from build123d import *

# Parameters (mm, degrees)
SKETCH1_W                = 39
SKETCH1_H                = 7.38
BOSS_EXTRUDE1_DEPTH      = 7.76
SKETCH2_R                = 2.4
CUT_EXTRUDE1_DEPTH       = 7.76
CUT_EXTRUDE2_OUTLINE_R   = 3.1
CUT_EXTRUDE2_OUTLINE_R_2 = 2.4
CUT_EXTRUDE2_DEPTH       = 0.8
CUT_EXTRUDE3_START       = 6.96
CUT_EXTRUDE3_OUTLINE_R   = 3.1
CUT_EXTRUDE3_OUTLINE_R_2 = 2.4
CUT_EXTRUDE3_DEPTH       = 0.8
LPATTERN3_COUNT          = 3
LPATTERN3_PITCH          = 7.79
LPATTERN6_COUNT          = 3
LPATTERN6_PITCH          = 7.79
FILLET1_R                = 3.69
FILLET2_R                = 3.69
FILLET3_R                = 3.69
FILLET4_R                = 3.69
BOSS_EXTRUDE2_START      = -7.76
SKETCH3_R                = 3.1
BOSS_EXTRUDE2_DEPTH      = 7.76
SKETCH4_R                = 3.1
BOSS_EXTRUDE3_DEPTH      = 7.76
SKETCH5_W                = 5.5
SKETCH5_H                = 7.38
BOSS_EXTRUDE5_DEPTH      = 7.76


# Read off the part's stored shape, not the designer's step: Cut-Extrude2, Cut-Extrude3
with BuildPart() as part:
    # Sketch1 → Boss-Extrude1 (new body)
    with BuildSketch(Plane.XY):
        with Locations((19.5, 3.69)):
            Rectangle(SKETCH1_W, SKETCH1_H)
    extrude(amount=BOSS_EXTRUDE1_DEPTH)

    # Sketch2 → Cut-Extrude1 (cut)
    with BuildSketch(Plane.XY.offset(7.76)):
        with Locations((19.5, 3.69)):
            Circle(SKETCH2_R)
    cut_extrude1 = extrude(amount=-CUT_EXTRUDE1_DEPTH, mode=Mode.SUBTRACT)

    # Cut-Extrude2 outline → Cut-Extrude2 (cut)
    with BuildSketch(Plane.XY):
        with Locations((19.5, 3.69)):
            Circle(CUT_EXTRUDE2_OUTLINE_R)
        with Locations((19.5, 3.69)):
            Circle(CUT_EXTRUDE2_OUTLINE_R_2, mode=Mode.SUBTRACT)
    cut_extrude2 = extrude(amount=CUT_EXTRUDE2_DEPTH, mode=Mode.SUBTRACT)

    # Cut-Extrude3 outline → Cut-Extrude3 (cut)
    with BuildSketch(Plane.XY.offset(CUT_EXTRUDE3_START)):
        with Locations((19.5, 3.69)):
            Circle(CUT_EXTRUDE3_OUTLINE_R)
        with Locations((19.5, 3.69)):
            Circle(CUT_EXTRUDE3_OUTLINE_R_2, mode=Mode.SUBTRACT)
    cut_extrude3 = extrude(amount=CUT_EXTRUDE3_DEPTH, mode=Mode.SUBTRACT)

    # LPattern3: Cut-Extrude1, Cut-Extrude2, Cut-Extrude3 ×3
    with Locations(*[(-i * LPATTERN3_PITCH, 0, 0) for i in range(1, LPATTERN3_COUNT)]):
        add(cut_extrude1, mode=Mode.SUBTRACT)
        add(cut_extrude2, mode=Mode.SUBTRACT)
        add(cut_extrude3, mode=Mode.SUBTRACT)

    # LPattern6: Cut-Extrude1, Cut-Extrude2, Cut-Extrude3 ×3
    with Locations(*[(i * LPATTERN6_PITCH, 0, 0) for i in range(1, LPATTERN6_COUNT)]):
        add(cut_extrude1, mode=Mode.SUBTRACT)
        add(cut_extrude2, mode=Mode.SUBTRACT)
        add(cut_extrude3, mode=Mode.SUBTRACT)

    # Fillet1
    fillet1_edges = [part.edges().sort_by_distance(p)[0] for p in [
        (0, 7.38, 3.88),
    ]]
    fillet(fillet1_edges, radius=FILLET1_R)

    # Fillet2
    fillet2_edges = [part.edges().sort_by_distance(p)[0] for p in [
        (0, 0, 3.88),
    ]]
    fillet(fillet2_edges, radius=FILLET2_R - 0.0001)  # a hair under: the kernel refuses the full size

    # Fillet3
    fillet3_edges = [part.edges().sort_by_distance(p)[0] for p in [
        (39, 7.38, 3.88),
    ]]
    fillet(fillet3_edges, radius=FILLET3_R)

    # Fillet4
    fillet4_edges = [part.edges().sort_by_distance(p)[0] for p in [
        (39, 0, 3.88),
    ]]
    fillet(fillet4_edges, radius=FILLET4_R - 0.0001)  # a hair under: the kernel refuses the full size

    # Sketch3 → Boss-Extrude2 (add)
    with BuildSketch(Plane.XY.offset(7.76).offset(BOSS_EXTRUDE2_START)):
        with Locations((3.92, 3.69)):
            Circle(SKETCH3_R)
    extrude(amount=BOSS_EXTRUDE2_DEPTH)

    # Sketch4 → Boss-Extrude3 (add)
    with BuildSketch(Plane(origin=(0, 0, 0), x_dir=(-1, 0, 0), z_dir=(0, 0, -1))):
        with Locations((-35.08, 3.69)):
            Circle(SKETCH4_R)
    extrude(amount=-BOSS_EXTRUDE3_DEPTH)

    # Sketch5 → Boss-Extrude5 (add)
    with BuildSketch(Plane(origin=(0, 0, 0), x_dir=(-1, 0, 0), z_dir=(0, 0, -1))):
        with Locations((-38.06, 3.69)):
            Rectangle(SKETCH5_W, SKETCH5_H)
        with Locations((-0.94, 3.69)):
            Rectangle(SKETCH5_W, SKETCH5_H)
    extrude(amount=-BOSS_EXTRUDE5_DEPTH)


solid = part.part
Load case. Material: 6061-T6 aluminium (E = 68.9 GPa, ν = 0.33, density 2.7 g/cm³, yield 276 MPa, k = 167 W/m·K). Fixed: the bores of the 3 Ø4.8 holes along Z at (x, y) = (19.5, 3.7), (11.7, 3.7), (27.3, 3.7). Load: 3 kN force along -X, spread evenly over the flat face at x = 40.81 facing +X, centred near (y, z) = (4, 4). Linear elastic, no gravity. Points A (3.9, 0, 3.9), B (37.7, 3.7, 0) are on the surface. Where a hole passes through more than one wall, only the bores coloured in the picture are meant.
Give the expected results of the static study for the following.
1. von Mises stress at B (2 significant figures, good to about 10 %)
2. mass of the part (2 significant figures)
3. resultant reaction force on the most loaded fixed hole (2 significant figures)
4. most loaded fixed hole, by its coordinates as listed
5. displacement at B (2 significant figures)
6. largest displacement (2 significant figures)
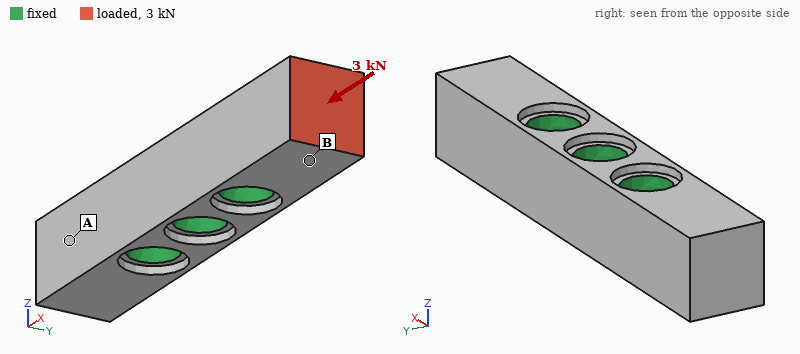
52 MPa
5.3 g
2.9 kN
(27.3, 3.7)
7.2 µm
9.6 µm
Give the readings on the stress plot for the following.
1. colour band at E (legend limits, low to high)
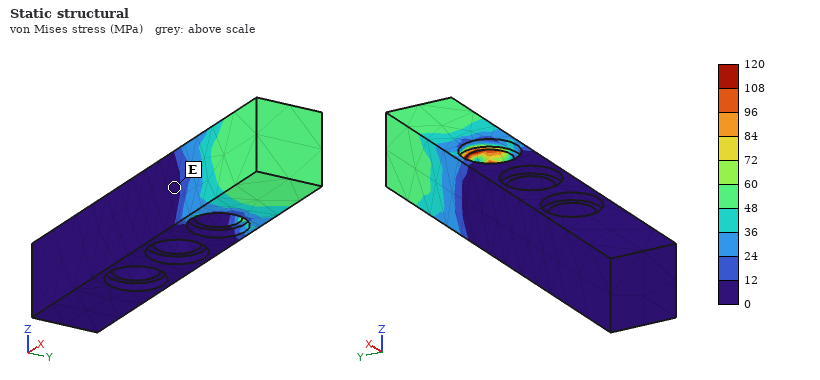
0 to 12 MPa
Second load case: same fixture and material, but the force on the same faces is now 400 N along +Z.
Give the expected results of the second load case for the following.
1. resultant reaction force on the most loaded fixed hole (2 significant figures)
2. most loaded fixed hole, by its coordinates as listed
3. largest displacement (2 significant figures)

420 N
(27.3, 3.7)
20 µm
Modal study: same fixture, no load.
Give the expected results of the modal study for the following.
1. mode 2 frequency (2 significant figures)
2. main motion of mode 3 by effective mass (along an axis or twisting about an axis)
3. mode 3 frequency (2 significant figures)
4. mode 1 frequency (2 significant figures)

29 kHz
along Z
31 kHz
29 kHz
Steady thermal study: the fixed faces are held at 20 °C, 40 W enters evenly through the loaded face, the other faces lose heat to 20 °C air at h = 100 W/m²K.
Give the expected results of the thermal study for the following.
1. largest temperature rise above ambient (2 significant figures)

50 K
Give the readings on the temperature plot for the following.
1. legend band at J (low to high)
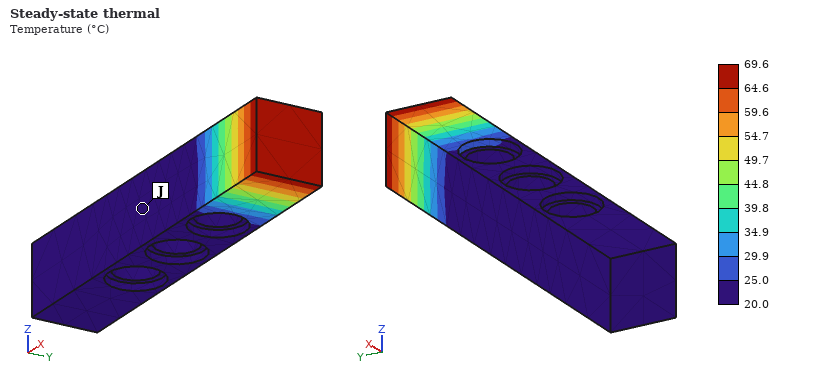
20.0 to 25.0 °C
